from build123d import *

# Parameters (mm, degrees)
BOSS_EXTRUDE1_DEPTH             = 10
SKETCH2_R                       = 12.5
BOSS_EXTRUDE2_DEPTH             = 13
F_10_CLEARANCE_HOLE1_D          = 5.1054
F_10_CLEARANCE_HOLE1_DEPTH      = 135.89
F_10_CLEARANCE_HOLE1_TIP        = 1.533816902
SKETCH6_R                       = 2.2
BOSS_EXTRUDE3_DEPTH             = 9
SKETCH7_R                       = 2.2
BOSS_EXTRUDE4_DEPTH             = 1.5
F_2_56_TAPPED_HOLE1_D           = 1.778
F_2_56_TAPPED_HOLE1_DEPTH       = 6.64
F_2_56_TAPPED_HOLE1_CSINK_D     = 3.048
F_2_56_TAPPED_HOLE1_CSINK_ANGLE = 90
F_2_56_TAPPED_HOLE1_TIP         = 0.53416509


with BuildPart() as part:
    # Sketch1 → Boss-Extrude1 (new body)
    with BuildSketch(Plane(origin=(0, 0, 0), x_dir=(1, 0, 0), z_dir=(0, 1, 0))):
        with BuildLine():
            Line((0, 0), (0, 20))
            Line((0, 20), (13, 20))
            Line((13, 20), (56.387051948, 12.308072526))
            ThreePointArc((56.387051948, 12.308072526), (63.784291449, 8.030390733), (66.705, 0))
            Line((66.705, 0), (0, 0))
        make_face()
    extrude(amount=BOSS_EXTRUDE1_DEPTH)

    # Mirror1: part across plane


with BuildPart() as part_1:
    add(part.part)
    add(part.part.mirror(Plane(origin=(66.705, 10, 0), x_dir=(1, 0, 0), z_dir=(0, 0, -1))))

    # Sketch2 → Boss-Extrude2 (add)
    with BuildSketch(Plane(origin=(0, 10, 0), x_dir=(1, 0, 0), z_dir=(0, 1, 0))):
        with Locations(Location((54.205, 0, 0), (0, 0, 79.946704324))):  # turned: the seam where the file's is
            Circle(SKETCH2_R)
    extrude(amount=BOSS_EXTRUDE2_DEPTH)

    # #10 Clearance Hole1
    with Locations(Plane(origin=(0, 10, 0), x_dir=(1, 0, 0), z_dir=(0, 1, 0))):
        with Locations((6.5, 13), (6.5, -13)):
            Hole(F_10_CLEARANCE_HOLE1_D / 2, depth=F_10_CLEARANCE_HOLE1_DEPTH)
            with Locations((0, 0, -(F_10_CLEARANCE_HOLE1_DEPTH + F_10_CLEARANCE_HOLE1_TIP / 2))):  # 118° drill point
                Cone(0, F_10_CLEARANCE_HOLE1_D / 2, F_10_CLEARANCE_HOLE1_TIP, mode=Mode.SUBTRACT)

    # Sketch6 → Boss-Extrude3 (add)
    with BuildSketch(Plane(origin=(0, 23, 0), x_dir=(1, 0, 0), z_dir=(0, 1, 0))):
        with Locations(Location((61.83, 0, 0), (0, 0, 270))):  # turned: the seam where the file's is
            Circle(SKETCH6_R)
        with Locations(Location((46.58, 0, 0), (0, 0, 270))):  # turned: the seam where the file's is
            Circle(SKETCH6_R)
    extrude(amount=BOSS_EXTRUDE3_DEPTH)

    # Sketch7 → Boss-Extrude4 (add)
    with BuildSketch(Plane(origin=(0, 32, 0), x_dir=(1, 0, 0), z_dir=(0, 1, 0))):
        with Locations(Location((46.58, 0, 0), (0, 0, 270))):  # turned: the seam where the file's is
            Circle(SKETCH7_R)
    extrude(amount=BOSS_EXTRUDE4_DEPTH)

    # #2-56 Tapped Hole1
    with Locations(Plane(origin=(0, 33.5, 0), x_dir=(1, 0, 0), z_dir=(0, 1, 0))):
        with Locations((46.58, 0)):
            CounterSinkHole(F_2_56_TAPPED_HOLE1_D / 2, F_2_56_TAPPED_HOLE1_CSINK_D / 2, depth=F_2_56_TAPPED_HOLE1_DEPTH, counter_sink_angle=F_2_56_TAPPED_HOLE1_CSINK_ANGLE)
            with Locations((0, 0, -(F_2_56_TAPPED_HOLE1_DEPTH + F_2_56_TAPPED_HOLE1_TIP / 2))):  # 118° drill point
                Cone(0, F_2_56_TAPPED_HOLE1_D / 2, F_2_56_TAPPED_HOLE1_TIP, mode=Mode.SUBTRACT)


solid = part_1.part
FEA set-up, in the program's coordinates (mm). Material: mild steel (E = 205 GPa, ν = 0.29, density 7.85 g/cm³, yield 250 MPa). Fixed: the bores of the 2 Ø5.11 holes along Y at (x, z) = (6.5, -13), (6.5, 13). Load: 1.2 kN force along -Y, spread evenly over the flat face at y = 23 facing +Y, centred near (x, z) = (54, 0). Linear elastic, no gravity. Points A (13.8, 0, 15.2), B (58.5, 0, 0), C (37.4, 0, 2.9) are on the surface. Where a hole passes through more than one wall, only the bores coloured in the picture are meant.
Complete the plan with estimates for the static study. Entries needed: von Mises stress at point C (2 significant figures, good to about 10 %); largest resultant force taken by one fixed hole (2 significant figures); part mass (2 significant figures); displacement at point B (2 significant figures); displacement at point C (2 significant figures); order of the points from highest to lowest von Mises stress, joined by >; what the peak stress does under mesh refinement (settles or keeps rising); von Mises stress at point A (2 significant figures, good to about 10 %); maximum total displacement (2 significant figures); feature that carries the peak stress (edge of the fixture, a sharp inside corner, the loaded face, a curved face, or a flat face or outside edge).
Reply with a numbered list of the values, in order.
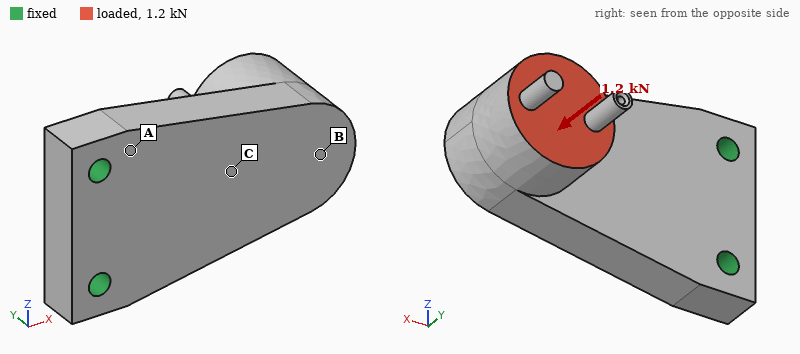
1. 39 MPa
2. 600 N
3. 210 g
4. 0.085 mm
5. 0.039 mm
6. A > C > B
7. keeps rising
8. 84 MPa
9. 0.12 mm
10. edge of the fixture
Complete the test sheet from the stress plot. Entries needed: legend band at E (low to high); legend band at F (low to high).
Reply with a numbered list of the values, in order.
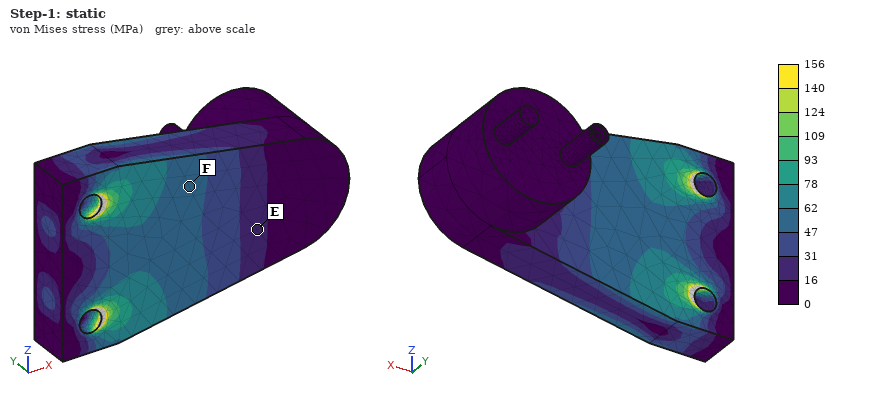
1. 16 to 31 MPa
2. 47 to 62 MPa
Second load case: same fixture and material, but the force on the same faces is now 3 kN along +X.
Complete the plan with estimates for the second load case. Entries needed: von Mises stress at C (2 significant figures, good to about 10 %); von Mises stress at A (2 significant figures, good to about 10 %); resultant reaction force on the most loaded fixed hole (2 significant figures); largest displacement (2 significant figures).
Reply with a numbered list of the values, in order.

1. 90 MPa
2. 82 MPa
3. 1.5 kN
4. 0.18 mm
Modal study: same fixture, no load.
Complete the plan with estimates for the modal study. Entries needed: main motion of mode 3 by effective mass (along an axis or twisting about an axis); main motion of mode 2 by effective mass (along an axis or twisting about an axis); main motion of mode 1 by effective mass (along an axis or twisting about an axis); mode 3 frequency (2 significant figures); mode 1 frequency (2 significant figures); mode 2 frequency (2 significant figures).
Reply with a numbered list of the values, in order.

1. along Z
2. along Z
3. along Y
4. 8600 Hz
5. 1900 Hz
6. 5200 Hz
